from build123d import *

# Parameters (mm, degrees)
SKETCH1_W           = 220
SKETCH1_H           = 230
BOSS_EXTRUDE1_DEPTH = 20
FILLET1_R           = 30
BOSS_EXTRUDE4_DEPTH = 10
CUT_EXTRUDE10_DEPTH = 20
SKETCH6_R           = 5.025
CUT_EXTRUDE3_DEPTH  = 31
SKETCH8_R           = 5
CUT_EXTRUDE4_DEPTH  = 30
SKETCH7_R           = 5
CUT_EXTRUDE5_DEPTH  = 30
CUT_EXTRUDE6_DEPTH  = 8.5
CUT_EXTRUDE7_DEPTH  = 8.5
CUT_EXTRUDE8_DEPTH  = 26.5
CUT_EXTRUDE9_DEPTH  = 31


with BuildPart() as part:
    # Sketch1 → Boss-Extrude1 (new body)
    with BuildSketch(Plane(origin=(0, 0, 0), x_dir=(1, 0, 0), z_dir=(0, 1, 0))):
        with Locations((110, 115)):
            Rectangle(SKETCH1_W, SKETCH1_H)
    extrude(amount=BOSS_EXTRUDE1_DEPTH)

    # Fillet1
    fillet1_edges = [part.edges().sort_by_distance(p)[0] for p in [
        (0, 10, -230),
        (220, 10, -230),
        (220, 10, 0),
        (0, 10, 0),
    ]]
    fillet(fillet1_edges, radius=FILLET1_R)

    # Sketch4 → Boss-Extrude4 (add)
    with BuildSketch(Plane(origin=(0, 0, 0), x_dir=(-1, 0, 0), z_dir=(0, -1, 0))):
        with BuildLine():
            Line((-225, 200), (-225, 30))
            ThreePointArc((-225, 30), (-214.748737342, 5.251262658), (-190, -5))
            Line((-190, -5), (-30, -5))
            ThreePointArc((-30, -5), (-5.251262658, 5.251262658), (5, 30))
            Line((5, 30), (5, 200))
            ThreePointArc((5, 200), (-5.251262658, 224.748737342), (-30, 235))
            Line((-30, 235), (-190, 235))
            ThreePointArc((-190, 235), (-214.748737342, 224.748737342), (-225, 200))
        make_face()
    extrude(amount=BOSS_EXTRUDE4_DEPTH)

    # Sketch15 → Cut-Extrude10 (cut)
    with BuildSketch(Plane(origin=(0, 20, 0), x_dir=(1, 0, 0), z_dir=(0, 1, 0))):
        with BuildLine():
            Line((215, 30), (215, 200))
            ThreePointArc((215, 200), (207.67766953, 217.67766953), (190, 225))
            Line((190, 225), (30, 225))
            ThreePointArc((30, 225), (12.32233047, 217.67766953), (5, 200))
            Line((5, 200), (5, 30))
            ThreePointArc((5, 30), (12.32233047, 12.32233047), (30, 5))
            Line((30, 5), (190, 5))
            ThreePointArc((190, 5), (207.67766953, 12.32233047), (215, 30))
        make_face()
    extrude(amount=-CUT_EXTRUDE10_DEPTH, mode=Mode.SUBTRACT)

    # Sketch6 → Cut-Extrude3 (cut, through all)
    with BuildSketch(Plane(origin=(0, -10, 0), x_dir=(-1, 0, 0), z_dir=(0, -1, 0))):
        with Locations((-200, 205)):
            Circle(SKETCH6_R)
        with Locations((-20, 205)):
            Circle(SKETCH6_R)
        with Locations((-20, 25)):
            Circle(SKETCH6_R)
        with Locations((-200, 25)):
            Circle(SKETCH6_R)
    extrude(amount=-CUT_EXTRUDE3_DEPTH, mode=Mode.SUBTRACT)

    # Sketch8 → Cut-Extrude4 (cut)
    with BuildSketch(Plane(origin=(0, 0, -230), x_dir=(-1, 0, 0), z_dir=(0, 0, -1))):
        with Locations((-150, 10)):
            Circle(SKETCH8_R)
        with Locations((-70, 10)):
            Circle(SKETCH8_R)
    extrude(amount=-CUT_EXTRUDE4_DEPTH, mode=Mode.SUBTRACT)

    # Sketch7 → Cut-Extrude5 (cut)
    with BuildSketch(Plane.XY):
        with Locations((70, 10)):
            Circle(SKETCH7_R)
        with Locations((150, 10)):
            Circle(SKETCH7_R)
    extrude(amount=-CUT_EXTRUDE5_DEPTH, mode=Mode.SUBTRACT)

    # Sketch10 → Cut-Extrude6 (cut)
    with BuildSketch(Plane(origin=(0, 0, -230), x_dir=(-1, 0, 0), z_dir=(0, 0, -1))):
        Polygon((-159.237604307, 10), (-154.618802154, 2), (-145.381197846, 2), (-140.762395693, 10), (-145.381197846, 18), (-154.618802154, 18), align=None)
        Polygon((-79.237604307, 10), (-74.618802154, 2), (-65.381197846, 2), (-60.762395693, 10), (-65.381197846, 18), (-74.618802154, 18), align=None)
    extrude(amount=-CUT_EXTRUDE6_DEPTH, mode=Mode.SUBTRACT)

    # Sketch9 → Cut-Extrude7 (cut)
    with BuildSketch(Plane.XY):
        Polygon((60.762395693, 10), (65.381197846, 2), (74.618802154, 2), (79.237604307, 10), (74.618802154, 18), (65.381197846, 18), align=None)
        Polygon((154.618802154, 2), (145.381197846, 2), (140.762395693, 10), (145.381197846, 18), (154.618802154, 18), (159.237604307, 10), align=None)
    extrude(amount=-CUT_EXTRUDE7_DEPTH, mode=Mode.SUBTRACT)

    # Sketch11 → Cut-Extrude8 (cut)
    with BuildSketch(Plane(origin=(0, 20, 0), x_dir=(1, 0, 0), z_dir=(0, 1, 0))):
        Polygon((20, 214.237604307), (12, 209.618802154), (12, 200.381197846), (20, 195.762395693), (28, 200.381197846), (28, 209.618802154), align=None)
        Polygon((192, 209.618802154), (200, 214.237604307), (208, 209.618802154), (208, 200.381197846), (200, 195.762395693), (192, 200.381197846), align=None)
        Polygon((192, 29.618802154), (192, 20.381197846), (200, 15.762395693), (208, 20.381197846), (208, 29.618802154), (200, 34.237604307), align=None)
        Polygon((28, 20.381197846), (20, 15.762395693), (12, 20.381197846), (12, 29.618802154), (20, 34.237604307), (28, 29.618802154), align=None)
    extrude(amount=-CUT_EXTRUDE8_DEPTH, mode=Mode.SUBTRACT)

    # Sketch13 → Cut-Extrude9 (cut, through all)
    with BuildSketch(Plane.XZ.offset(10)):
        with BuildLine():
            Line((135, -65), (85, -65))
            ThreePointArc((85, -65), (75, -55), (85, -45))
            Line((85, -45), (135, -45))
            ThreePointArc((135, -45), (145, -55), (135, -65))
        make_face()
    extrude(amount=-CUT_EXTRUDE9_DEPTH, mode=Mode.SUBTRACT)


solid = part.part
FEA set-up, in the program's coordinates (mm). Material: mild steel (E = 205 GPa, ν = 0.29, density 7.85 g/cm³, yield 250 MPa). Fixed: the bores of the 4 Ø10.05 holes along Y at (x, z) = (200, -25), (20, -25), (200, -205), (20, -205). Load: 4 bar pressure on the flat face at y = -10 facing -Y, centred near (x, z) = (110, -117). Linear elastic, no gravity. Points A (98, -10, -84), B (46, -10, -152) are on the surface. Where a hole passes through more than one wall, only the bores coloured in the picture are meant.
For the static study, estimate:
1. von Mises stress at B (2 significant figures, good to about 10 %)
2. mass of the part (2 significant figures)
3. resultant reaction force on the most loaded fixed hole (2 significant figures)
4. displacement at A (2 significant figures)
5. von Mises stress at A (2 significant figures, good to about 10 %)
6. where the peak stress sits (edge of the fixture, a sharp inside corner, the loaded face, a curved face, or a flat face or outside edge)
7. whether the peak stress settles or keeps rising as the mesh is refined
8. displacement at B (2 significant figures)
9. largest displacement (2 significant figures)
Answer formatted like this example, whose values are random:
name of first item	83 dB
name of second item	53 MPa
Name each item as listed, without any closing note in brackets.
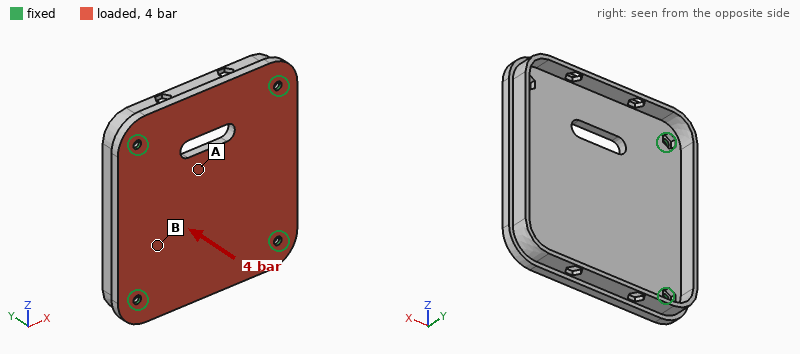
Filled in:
von Mises stress at B	21 MPa
mass of the part	4.7 kg
resultant reaction force on the most loaded fixed hole	8.8 kN
displacement at A	0.18 mm
von Mises stress at A	41 MPa
where the peak stress sits	edge of the fixture
whether the peak stress settles or keeps rising as the mesh is refined	keeps rising
displacement at B	0.10 mm
largest displacement	0.19 mm
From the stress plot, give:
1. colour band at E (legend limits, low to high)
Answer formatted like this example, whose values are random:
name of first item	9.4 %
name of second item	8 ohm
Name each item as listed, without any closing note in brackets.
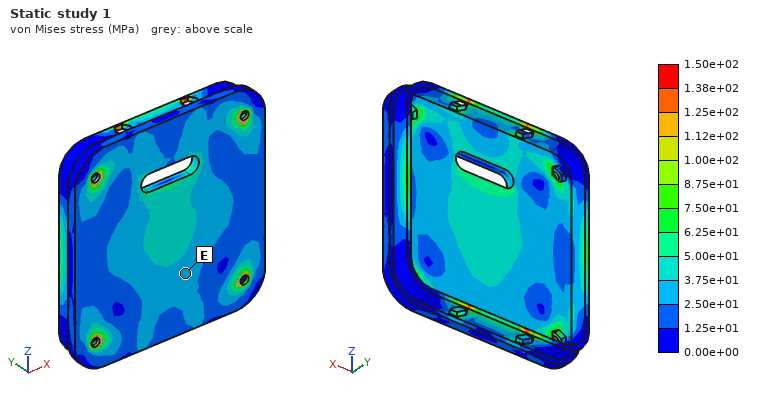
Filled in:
colour band at E	2.50e+01 to 3.75e+01 MPa
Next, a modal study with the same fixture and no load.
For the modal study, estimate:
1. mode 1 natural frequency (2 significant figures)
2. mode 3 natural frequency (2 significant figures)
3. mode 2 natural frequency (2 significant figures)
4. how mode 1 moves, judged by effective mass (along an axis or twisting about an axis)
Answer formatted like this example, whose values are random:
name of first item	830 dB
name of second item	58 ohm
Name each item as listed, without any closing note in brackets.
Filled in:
mode 1 natural frequency	1000 Hz
mode 3 natural frequency	1700 Hz
mode 2 natural frequency	1700 Hz
how mode 1 moves, judged by effective mass	along Y
